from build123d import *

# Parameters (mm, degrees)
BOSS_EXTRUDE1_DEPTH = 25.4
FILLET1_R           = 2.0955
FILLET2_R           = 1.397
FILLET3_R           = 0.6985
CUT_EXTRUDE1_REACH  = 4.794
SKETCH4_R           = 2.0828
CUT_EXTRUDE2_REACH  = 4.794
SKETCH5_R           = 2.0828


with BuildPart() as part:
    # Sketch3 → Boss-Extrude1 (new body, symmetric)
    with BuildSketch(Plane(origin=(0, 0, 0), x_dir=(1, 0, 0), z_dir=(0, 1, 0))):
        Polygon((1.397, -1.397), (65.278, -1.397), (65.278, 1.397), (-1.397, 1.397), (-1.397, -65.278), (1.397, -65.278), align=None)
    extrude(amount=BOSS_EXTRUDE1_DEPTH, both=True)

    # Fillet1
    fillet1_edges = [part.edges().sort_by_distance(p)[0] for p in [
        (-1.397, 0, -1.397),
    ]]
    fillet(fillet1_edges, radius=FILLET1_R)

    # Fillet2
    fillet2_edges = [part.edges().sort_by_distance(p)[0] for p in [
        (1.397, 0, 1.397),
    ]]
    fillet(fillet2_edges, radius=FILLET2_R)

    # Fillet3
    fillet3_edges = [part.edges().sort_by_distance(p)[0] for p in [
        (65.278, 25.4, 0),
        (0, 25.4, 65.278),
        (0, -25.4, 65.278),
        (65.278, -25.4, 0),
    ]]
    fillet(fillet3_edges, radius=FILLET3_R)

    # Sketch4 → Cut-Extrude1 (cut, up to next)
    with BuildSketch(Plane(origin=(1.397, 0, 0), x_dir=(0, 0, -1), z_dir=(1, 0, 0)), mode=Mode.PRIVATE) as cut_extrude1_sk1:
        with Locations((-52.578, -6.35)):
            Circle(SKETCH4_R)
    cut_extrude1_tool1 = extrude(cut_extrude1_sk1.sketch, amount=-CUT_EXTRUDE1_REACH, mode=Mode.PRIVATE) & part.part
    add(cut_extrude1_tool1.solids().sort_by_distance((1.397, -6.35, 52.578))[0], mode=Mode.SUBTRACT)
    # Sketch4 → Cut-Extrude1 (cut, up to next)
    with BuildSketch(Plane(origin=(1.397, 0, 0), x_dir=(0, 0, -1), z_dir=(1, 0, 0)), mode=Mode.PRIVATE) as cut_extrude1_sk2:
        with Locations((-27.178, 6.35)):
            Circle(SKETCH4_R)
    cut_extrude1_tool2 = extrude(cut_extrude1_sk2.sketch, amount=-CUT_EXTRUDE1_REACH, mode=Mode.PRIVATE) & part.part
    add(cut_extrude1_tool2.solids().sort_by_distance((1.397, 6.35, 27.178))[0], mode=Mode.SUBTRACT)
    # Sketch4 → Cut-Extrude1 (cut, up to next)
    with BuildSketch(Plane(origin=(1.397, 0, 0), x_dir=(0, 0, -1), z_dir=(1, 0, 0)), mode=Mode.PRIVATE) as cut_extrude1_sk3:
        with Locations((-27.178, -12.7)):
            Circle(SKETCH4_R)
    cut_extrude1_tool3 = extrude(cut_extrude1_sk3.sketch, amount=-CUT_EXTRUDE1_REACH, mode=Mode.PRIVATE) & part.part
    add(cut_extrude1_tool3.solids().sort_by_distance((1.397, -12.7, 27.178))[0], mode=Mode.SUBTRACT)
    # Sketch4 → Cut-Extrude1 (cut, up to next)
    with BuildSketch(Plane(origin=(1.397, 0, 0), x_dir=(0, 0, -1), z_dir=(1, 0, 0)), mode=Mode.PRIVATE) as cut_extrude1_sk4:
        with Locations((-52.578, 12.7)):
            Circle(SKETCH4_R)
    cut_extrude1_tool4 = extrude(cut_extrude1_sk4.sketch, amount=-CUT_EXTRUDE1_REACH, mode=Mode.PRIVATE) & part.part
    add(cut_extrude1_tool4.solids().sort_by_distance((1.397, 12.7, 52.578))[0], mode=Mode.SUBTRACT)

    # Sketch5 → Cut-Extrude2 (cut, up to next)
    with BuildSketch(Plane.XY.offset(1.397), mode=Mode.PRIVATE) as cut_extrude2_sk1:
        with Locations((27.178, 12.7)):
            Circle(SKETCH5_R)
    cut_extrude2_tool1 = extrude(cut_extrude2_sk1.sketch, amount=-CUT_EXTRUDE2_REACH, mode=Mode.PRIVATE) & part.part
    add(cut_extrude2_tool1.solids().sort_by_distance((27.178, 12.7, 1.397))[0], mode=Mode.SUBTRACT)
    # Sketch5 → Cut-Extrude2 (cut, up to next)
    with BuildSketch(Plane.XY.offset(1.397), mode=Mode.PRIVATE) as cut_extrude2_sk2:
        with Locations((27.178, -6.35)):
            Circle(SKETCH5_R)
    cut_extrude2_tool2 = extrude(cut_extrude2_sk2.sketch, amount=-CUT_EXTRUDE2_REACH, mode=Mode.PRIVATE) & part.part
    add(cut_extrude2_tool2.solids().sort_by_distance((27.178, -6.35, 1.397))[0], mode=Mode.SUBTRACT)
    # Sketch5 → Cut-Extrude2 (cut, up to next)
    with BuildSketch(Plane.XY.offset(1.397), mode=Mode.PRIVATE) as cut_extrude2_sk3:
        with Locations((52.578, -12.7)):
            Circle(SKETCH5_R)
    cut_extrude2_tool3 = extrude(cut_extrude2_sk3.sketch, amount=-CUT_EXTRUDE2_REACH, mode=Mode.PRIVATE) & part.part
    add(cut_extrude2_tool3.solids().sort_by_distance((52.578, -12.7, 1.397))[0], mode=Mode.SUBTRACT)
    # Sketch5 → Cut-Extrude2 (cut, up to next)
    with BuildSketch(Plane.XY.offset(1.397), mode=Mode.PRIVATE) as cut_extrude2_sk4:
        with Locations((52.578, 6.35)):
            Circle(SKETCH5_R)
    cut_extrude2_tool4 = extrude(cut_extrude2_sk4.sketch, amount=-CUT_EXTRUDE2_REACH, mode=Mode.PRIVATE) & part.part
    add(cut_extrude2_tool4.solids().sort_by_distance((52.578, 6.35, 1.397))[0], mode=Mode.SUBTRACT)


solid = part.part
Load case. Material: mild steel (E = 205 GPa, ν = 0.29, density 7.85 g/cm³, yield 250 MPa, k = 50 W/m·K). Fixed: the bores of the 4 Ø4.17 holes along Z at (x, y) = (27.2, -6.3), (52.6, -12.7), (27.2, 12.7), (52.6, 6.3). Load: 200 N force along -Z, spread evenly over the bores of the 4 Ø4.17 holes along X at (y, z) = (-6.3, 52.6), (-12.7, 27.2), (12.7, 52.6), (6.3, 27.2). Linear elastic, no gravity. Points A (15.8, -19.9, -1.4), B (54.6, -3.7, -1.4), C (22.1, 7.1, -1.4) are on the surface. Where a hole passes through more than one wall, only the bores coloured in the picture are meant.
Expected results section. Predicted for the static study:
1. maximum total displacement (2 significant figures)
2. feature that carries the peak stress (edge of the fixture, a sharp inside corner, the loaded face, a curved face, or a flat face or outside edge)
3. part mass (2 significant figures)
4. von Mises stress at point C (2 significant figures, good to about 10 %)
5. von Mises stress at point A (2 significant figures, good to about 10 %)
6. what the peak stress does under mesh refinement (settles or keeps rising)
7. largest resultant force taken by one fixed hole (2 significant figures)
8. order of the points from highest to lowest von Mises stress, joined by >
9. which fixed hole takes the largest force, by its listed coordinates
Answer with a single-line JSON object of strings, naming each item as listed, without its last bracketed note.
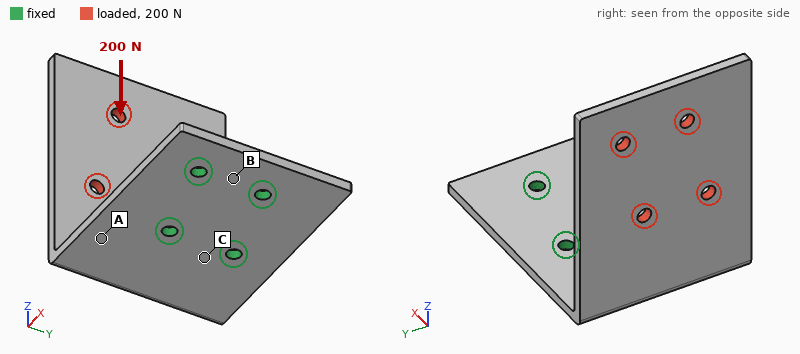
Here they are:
{"maximum total displacement": "0.26 mm", "feature that carries the peak stress": "edge of the fixture", "part mass": "140 g", "von Mises stress at point C": "62 MPa", "von Mises stress at point A": "41 MPa", "what the peak stress does under mesh refinement": "keeps rising", "largest resultant force taken by one fixed hole": "160 N", "order of the points from highest to lowest von Mises stress, joined by >": "C > A > B", "which fixed hole takes the largest force, by its listed coordinates": "(27.2, -6.3)"}
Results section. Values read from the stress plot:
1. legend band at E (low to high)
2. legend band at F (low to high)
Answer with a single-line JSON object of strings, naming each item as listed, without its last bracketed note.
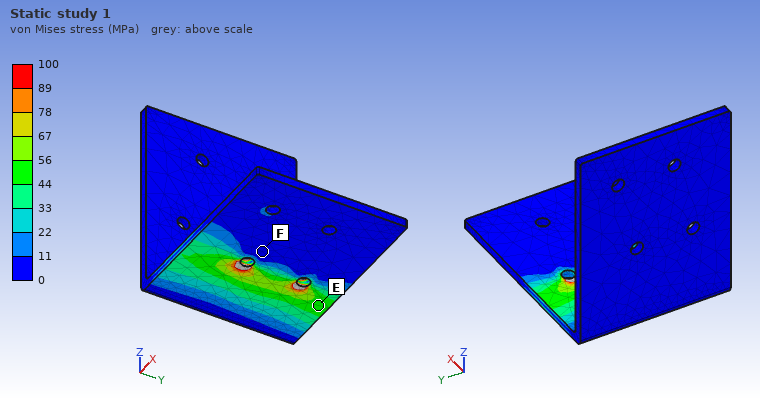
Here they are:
{"legend band at E": "44 to 56 MPa", "legend band at F": "0 to 11 MPa"}
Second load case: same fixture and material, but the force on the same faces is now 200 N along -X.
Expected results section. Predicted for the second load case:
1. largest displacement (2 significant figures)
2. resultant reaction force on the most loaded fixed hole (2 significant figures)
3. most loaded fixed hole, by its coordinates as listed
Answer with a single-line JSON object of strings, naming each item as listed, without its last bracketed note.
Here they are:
{"largest displacement": "1.1 mm", "resultant reaction force on the most loaded fixed hole": "120 N", "most loaded fixed hole, by its coordinates as listed": "(27.2, -6.3)"}
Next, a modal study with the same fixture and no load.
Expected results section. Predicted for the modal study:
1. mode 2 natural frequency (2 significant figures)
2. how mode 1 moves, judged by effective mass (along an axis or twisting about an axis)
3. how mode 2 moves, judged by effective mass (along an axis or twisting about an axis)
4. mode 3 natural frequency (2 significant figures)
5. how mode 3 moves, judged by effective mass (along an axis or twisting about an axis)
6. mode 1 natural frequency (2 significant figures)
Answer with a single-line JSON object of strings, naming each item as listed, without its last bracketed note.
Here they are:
{"mode 2 natural frequency": "650 Hz", "how mode 1 moves, judged by effective mass": "along X", "how mode 2 moves, judged by effective mass": "along Y", "mode 3 natural frequency": "1300 Hz", "how mode 3 moves, judged by effective mass": "along Z", "mode 1 natural frequency": "340 Hz"}
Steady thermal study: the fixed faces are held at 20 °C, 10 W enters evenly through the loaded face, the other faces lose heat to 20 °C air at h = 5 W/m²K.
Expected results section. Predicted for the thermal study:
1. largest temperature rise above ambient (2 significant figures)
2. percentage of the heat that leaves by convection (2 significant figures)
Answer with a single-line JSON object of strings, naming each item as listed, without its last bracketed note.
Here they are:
{"largest temperature rise above ambient": "81 K", "percentage of the heat that leaves by convection": "24 %"}
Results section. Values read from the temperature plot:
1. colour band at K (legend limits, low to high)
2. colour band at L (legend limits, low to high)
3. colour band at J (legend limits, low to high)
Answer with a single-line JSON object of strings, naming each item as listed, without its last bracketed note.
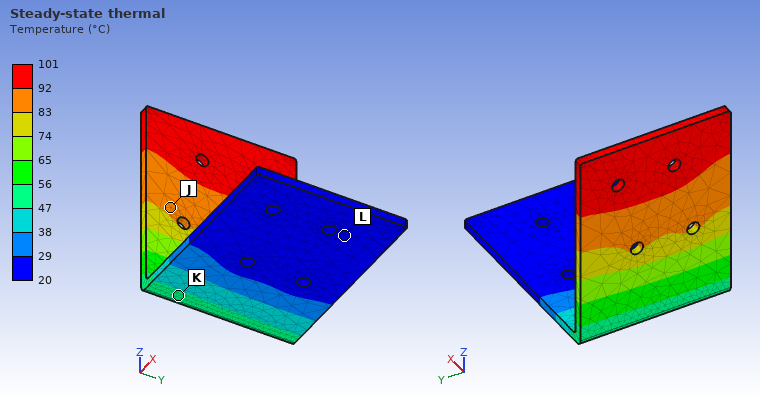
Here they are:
{"colour band at K": "47 to 56 °C", "colour band at L": "20 to 29 °C", "colour band at J": "83 to 92 °C"}
